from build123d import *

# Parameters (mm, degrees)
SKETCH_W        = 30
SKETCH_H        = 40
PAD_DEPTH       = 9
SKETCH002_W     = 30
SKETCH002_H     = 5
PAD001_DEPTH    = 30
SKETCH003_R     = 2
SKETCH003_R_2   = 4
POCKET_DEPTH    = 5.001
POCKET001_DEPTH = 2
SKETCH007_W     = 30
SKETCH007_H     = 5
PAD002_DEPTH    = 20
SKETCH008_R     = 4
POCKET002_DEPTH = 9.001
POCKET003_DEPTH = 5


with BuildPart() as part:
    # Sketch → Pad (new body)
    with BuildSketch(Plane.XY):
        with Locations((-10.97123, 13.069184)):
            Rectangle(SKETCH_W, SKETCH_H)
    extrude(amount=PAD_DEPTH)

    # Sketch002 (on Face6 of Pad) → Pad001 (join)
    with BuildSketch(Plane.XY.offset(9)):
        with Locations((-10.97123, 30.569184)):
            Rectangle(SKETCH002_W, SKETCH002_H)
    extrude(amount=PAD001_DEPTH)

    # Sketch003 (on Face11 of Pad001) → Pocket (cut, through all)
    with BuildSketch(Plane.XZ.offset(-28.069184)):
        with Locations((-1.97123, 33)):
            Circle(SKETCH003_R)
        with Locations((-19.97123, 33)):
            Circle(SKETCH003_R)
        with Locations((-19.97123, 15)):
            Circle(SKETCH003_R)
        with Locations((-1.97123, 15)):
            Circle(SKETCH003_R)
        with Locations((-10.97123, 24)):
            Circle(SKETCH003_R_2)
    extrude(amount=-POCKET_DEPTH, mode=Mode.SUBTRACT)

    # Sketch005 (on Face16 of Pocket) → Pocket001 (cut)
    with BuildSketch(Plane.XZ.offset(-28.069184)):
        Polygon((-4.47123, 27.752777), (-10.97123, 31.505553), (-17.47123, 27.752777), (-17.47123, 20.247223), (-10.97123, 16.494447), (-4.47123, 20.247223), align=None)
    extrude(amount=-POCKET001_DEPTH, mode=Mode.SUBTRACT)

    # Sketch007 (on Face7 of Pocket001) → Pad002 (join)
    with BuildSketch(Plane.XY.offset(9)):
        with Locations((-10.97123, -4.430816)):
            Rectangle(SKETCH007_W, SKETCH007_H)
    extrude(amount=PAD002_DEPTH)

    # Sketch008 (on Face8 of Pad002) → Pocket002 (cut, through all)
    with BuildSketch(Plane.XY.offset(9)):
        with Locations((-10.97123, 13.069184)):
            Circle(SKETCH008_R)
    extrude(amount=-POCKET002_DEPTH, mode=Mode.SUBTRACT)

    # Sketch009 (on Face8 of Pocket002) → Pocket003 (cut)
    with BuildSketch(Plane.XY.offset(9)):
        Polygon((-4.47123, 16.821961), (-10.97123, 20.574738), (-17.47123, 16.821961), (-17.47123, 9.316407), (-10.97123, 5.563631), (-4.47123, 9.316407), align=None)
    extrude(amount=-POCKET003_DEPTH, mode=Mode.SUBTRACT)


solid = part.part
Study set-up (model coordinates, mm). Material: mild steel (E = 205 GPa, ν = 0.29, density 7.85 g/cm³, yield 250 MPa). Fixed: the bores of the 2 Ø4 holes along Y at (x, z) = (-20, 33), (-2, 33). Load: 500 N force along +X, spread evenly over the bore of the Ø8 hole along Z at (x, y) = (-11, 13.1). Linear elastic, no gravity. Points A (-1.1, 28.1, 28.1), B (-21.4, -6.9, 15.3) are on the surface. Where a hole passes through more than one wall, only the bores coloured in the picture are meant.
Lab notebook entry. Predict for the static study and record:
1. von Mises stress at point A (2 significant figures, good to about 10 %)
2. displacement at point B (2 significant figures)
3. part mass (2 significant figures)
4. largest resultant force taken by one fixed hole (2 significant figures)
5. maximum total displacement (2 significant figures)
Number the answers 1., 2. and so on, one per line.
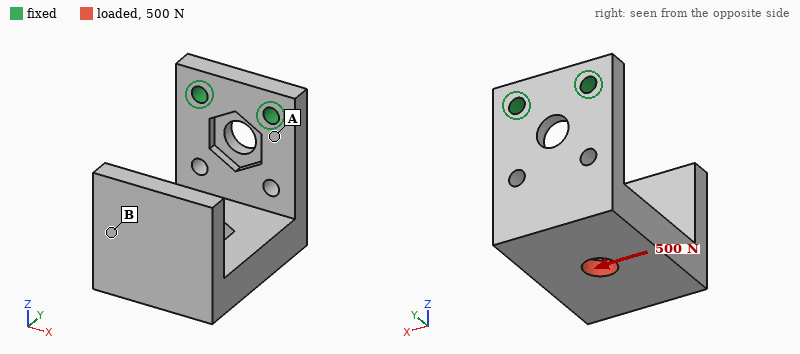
1. 65 MPa
2. 76 µm
3. 130 g
4. 800 N
5. 79 µm
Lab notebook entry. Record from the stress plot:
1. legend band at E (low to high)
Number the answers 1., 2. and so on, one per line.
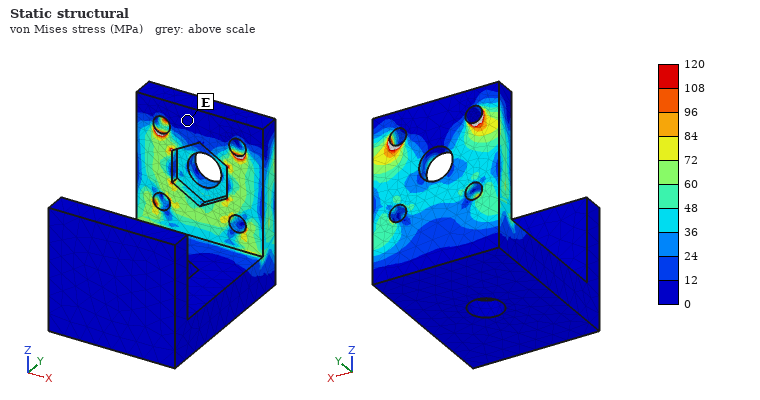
1. 0 to 12 MPa
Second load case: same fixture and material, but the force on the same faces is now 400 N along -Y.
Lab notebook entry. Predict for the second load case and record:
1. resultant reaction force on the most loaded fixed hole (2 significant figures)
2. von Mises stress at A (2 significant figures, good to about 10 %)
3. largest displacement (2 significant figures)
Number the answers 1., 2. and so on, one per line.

1. 210 N
2. 130 MPa
3. 0.18 mm
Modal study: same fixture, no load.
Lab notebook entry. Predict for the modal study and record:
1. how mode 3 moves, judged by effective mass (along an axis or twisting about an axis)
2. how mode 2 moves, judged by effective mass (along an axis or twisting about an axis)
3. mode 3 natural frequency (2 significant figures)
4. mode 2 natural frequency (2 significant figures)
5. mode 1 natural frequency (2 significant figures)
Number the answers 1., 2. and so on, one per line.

1. along Y
2. along X
3. 2600 Hz
4. 1200 Hz
5. 720 Hz
